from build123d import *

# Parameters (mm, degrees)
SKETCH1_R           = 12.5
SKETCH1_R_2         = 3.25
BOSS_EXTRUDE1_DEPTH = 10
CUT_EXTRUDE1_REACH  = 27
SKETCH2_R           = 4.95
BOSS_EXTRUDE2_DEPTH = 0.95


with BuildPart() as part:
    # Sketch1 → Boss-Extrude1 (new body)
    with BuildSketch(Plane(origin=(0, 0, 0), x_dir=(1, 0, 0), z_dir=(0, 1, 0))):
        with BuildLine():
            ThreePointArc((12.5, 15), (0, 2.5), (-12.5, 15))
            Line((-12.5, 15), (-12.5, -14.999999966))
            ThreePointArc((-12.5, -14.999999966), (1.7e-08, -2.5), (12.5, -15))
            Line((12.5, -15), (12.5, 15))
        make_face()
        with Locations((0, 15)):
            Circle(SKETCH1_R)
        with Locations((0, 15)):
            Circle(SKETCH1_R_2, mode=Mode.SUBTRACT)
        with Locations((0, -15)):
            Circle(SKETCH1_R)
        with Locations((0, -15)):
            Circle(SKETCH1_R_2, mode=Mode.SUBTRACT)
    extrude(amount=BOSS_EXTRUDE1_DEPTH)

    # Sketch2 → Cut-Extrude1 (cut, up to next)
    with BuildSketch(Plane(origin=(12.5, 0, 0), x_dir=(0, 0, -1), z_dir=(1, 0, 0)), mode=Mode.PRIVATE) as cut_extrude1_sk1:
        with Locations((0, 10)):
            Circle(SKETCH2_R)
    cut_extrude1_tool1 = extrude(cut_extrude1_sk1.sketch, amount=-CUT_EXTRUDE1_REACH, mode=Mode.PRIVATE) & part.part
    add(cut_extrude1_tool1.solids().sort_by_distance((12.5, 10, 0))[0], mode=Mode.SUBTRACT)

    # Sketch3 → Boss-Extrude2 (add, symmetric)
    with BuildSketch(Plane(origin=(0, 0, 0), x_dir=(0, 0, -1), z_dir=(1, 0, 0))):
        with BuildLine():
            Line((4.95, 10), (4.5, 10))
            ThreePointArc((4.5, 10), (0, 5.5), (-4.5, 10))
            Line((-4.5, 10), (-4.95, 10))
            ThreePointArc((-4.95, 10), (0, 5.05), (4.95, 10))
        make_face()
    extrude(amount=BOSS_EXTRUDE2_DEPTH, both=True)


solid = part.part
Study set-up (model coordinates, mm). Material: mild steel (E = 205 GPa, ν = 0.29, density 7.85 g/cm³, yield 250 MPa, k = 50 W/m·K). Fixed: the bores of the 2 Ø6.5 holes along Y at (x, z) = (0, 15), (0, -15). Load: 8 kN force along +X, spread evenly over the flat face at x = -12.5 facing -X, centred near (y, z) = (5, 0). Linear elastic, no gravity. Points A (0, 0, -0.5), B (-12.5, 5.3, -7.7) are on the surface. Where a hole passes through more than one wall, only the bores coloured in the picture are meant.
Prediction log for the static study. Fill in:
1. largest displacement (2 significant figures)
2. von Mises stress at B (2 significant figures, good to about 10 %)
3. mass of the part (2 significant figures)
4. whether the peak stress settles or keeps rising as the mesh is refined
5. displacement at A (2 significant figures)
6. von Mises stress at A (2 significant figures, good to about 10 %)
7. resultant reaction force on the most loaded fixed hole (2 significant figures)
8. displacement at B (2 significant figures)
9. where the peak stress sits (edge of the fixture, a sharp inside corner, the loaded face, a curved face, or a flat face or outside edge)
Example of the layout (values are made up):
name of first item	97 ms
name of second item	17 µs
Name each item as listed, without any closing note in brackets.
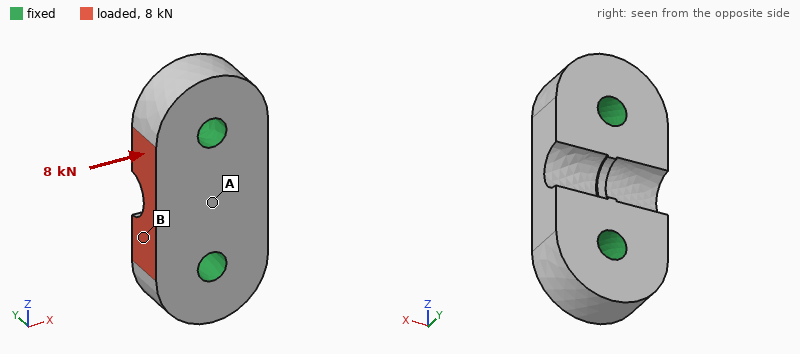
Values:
largest displacement	4.0 µm
von Mises stress at B	29 MPa
mass of the part	85 g
whether the peak stress settles or keeps rising as the mesh is refined	keeps rising
displacement at A	2.5 µm
von Mises stress at A	15 MPa
resultant reaction force on the most loaded fixed hole	4.1 kN
displacement at B	2.9 µm
where the peak stress sits	edge of the fixture
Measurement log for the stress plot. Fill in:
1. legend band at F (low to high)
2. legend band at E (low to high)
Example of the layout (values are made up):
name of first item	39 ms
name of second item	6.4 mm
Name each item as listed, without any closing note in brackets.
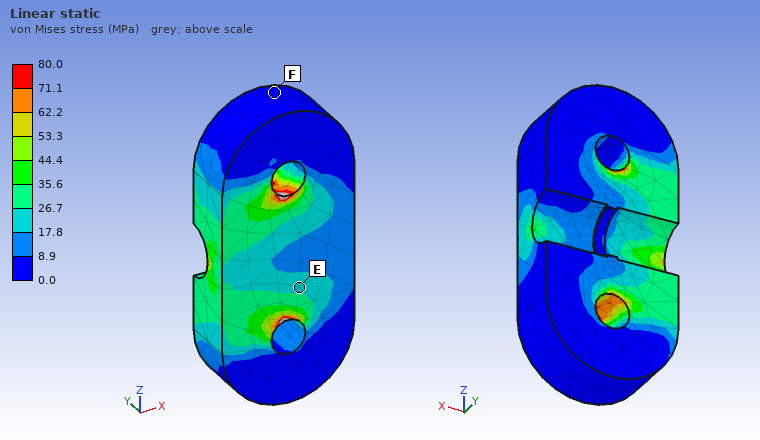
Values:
legend band at F	0.0 to 8.9 MPa
legend band at E	17.8 to 26.7 MPa
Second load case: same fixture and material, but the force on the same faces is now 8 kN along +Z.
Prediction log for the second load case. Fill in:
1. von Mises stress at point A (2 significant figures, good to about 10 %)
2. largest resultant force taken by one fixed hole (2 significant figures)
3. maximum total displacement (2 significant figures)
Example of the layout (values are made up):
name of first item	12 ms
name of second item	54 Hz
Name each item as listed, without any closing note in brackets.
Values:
von Mises stress at point A	22 MPa
largest resultant force taken by one fixed hole	4.7 kN
maximum total displacement	5.7 µm
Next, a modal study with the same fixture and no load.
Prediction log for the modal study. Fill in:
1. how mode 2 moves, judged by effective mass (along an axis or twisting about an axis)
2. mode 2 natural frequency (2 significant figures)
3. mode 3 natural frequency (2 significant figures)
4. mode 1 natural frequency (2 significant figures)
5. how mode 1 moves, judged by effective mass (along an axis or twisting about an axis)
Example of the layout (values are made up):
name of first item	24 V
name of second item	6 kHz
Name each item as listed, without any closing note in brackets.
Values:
how mode 2 moves, judged by effective mass	along Y
mode 2 natural frequency	36 kHz
mode 3 natural frequency	42 kHz
mode 1 natural frequency	35 kHz
how mode 1 moves, judged by effective mass	twisting about Z
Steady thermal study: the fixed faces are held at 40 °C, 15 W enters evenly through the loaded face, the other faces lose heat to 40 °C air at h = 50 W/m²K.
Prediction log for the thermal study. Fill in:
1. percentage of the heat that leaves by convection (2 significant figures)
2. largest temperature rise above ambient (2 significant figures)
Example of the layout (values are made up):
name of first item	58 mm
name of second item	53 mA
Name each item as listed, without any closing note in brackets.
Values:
percentage of the heat that leaves by convection	3.0 %
largest temperature rise above ambient	13 K
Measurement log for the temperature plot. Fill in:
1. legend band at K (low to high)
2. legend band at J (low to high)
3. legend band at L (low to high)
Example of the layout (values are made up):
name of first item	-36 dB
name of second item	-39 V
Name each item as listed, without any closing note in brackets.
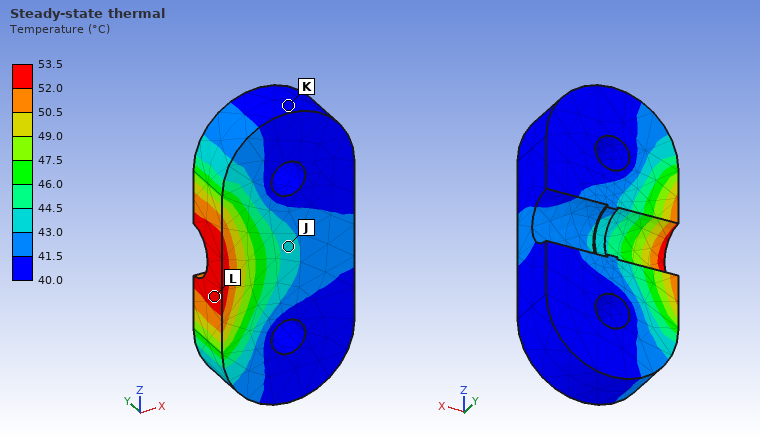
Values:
legend band at K	40.0 to 41.5 °C
legend band at J	43.0 to 44.5 °C
legend band at L	52.0 to 53.5 °C
